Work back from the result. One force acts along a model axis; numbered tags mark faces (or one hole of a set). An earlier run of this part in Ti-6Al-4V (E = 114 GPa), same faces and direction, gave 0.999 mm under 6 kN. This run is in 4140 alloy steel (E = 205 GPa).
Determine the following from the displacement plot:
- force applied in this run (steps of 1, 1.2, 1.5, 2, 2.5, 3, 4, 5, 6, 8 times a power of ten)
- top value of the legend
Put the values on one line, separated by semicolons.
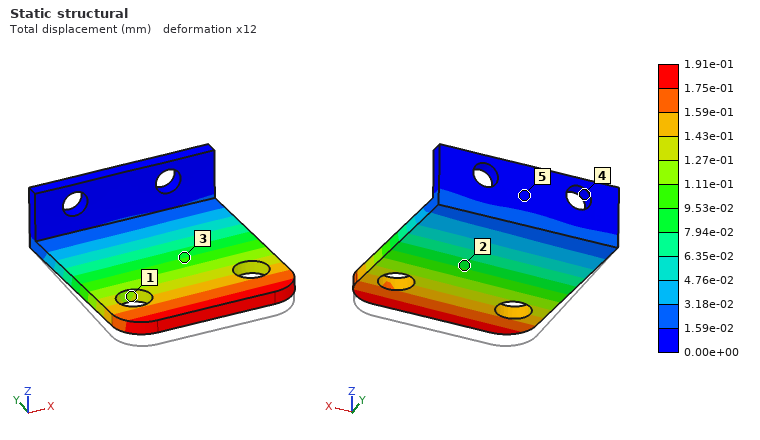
2 kN; 1.91e-01 mm
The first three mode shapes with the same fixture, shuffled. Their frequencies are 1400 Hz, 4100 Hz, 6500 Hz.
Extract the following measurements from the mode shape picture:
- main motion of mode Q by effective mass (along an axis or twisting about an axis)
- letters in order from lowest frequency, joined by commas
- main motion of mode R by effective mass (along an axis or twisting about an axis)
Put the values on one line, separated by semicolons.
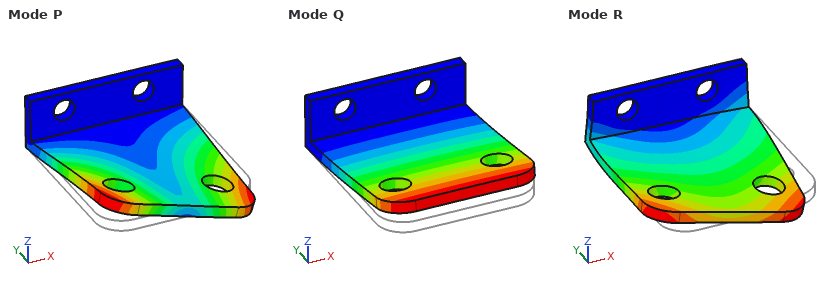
along Z; Q, P, R; along X
